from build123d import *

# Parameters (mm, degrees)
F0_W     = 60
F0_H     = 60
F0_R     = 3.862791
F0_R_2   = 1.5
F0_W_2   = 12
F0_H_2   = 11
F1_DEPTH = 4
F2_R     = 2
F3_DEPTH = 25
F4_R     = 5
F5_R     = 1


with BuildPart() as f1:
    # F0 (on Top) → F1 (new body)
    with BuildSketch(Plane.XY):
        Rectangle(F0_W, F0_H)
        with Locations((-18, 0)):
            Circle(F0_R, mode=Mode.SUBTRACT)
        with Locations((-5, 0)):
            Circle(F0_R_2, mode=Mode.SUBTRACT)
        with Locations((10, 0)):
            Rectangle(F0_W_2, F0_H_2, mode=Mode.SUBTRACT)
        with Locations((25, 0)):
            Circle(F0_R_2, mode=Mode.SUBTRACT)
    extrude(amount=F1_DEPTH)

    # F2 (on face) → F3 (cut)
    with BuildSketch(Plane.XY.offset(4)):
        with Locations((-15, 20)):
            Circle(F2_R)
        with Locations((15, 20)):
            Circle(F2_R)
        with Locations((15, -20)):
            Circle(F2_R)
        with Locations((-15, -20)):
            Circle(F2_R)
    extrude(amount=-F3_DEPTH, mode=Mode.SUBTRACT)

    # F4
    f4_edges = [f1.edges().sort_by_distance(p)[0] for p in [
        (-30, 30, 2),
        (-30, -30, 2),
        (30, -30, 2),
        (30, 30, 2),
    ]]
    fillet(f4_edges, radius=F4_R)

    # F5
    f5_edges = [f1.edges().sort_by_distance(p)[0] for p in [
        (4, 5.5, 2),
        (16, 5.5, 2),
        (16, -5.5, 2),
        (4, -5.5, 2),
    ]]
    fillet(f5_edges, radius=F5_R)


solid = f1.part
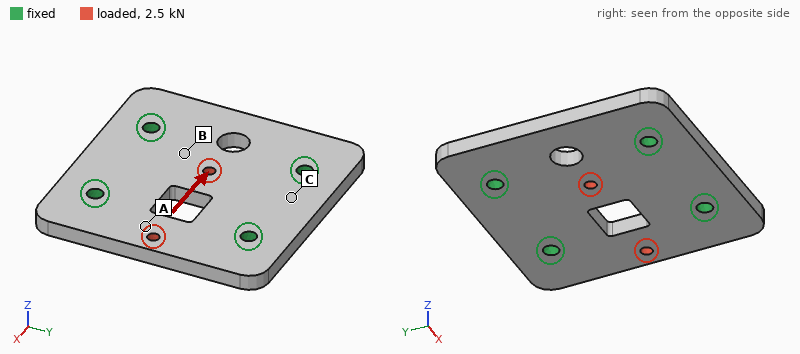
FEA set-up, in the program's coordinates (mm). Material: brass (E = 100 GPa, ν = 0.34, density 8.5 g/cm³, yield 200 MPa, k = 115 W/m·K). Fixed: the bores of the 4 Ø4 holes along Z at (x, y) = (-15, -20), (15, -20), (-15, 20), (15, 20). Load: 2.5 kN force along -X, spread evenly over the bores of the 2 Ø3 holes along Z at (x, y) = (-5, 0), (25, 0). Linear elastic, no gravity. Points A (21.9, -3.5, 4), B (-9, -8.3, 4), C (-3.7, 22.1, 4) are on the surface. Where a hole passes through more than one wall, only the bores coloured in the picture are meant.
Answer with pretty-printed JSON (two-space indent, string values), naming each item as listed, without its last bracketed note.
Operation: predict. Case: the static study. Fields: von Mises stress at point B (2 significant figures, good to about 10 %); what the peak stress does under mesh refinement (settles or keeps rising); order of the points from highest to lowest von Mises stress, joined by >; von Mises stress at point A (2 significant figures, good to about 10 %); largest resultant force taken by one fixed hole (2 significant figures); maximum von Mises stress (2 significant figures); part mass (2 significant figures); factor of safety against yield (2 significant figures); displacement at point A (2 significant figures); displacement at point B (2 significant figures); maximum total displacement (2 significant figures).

{
  "von Mises stress at point B": "11 MPa",
  "what the peak stress does under mesh refinement": "settles",
  "order of the points from highest to lowest von Mises stress, joined by >": "A > B > C",
  "von Mises stress at point A": "26 MPa",
  "largest resultant force taken by one fixed hole": "700 N",
  "maximum von Mises stress": "62 MPa",
  "part mass": "110 g",
  "factor of safety against yield": "3.2",
  "displacement at point A": "5.3 µm",
  "displacement at point B": "2.0 µm",
  "maximum total displacement": "7.4 µm"
}
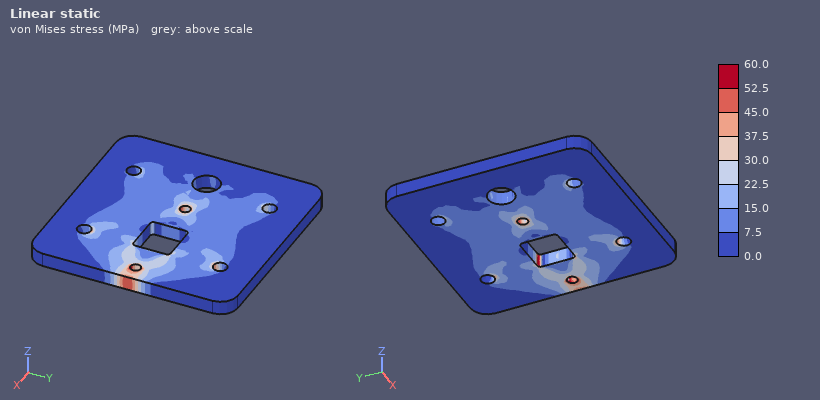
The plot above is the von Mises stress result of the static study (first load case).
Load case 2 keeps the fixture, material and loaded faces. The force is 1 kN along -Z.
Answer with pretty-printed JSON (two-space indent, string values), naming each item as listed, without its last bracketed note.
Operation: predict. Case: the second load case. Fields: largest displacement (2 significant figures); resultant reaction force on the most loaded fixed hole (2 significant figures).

{
  "largest displacement": "46 µm",
  "resultant reaction force on the most loaded fixed hole": "360 N"
}
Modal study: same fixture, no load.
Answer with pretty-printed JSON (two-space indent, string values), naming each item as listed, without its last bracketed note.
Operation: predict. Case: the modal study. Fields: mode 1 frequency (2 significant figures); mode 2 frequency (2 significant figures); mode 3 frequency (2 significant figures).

{
  "mode 1 frequency": "6600 Hz",
  "mode 2 frequency": "6700 Hz",
  "mode 3 frequency": "8000 Hz"
}
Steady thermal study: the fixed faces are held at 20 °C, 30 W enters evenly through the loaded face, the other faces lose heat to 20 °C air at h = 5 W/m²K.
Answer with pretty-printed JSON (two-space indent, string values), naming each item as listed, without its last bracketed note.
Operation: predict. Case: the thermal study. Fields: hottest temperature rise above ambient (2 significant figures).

{
  "hottest temperature rise above ambient": "27 K"
}
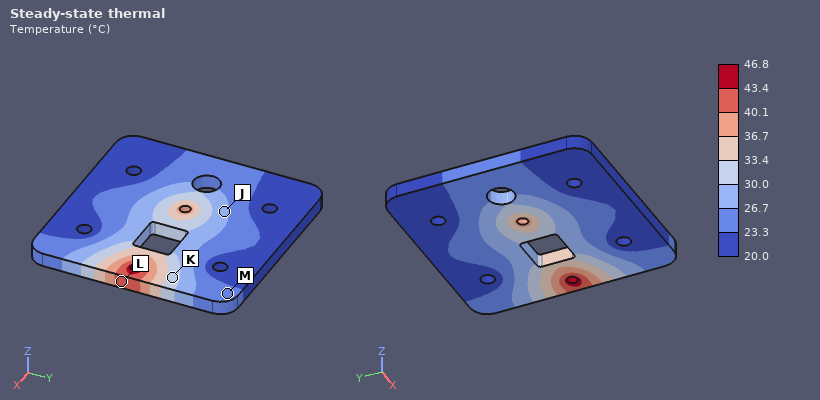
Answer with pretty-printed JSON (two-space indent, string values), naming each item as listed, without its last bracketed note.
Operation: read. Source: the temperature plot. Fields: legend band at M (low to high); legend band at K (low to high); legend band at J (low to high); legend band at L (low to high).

{
  "legend band at M": "23.3 to 26.7 °C",
  "legend band at K": "30.0 to 33.4 °C",
  "legend band at J": "26.7 to 30.0 °C",
  "legend band at L": "40.1 to 43.4 °C"
}
